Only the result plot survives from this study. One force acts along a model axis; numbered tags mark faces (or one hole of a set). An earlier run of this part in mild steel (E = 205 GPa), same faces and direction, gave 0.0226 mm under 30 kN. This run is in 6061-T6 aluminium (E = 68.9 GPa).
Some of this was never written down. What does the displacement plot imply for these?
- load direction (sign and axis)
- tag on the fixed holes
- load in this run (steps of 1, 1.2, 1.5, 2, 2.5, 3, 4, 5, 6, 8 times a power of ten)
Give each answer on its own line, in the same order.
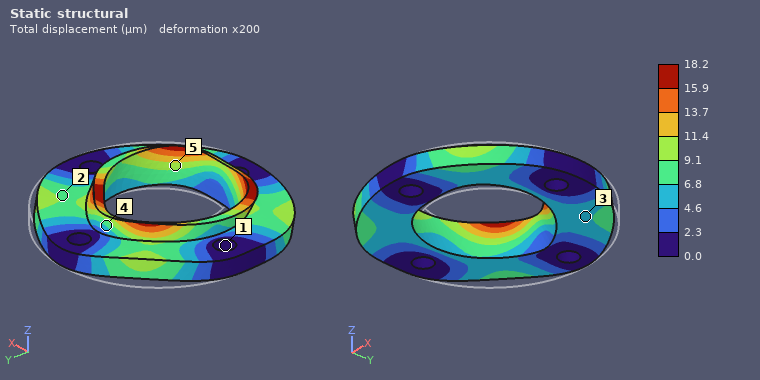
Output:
-Y
1
8 kN
